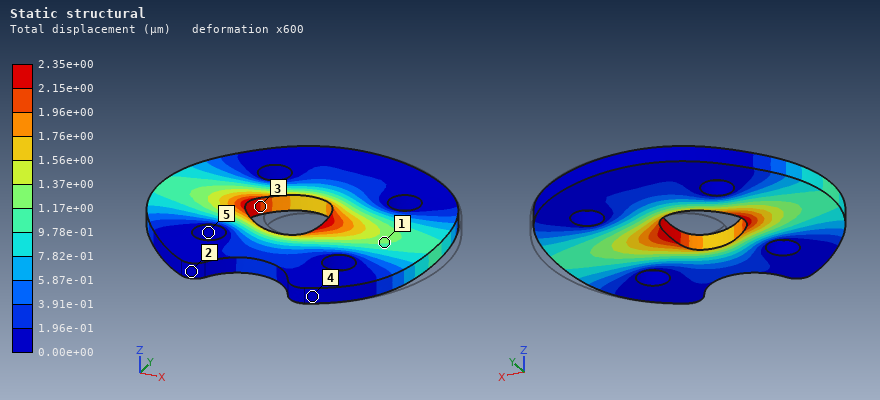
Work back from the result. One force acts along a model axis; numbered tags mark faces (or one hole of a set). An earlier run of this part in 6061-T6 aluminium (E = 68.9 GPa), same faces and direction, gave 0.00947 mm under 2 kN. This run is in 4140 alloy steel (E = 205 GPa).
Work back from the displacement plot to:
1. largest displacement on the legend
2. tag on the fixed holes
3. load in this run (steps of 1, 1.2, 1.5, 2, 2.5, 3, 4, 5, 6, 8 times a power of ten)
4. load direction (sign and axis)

2.35e+00 µm
5
1.5 kN
-X
